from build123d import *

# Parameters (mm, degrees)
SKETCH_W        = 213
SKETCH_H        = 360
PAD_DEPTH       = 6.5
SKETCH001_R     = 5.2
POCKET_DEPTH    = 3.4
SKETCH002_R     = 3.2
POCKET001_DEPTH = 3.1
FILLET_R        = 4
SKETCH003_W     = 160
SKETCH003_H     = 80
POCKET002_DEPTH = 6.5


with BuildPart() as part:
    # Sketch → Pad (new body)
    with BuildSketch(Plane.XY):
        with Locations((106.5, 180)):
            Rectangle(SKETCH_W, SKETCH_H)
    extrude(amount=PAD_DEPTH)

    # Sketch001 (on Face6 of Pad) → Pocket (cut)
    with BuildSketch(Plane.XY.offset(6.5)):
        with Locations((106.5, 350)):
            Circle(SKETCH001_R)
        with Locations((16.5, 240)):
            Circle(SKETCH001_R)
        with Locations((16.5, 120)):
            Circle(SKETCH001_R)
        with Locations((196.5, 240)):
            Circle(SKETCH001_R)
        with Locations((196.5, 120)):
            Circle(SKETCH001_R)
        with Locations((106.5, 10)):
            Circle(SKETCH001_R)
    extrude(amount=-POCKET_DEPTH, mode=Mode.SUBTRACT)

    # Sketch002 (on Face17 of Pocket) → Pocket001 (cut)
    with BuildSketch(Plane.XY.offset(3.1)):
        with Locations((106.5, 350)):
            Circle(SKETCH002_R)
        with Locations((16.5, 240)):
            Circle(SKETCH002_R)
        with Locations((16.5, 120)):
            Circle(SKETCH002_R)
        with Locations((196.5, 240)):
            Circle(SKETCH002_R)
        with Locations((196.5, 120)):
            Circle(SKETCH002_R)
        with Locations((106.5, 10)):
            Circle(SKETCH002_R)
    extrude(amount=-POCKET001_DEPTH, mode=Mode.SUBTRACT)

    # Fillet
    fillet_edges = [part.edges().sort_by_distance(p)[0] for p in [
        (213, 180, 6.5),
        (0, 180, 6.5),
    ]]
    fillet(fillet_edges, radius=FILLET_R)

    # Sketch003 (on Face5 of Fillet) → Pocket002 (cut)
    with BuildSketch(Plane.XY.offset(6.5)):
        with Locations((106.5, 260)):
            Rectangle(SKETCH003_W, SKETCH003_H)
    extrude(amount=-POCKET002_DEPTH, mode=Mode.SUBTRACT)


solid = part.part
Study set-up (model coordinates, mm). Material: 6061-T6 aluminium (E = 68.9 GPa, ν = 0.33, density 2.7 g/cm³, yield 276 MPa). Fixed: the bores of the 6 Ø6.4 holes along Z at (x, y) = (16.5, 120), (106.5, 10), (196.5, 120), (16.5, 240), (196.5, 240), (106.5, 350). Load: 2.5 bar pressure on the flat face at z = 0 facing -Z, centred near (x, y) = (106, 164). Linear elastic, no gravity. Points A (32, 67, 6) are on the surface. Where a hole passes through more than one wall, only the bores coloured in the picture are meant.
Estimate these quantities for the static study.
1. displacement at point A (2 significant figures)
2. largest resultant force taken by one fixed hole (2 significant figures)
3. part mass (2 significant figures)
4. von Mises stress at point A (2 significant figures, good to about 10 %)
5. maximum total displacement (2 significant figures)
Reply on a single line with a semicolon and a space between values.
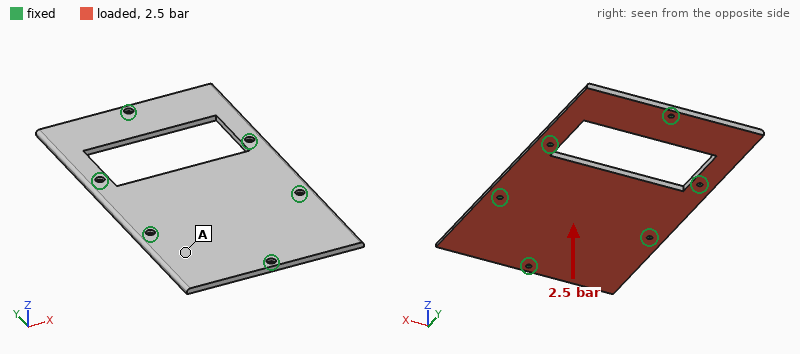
0.39 mm; 5.2 kN; 1.1 kg; 60 MPa; 1.3 mm
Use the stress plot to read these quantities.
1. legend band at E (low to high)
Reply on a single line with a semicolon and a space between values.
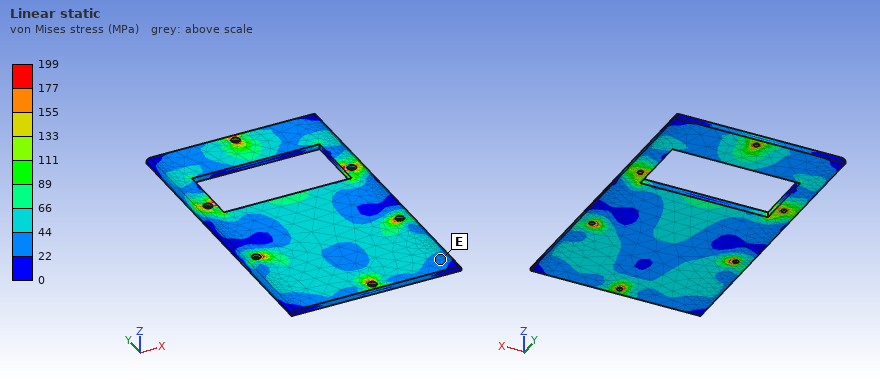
22 to 44 MPa
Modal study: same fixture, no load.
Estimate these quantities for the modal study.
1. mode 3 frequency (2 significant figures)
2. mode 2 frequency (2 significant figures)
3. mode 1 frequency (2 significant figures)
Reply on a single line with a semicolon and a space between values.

670 Hz; 670 Hz; 560 Hz
